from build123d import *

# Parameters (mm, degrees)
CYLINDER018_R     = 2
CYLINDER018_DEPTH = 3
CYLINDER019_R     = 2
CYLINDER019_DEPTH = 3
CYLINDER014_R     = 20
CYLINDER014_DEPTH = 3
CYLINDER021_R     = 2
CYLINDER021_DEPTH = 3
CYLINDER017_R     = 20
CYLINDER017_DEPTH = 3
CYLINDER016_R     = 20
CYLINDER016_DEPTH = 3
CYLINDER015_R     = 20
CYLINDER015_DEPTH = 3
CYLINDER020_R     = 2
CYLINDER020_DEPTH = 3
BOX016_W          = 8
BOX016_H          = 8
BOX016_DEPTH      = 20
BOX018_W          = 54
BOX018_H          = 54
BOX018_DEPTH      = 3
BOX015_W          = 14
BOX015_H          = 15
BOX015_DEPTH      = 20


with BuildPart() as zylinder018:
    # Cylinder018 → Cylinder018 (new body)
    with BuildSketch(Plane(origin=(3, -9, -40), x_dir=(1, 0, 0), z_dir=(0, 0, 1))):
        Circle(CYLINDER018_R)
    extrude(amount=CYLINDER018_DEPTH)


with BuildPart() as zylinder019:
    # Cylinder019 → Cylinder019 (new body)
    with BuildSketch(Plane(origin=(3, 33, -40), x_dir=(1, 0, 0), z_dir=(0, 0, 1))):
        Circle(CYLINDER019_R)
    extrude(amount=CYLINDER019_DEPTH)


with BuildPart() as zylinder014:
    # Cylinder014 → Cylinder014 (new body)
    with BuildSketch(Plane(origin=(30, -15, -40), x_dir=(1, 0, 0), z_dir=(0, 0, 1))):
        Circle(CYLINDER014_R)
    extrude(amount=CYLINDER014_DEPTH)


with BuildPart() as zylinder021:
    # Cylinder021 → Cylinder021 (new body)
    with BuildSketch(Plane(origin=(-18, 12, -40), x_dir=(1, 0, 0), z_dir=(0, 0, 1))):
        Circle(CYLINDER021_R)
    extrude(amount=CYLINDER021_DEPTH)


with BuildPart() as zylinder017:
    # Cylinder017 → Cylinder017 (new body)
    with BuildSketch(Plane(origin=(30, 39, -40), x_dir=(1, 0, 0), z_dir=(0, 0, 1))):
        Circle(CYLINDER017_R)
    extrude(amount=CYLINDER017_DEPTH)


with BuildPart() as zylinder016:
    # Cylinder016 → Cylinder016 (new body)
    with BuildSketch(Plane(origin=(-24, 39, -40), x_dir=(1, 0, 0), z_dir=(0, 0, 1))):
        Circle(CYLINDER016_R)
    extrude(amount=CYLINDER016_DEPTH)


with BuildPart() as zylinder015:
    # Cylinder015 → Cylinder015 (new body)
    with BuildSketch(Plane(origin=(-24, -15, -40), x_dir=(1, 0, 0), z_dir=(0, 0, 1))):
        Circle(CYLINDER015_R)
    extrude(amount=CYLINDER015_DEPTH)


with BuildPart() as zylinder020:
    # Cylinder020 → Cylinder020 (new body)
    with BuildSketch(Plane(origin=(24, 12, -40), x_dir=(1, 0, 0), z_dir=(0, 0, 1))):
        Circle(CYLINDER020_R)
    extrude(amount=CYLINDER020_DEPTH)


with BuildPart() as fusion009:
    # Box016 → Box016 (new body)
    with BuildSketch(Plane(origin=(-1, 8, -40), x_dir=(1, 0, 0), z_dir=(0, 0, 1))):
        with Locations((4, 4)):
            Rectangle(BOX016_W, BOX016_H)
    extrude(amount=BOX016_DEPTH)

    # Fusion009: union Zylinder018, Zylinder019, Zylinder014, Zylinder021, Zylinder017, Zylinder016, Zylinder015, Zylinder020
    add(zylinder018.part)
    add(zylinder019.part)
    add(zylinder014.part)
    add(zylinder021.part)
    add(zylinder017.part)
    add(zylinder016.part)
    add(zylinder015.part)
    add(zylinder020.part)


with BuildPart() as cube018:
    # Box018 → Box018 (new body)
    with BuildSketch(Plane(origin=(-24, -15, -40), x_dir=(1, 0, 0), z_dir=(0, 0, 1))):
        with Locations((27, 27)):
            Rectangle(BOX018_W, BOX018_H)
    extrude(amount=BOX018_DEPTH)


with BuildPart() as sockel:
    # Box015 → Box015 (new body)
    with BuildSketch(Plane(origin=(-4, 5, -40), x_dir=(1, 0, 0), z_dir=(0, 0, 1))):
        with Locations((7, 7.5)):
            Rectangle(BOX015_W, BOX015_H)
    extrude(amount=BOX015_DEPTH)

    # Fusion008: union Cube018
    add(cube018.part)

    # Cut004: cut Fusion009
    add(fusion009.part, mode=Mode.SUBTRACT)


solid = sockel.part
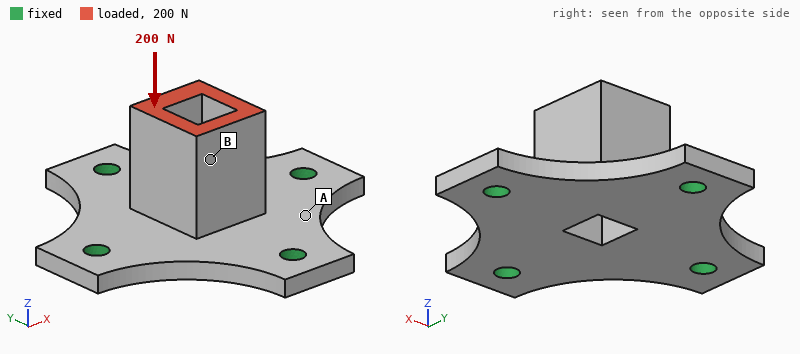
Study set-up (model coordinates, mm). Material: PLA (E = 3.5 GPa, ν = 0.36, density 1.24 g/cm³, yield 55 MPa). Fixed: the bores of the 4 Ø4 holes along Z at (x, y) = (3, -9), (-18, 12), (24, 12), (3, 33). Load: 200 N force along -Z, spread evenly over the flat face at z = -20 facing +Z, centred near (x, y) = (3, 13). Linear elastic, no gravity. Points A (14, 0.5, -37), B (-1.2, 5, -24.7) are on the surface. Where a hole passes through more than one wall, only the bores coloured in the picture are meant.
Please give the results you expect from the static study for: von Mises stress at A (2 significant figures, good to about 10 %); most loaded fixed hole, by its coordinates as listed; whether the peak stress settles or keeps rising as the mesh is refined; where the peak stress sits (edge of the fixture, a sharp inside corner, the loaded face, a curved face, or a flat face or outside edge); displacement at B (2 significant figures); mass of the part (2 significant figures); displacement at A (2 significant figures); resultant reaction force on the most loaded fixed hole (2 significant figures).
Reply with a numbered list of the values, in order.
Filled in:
1. 4.7 MPa
2. (3, 33)
3. keeps rising
4. edge of the fixture
5. 0.10 mm
6. 8.8 g
7. 0.046 mm
8. 59 N
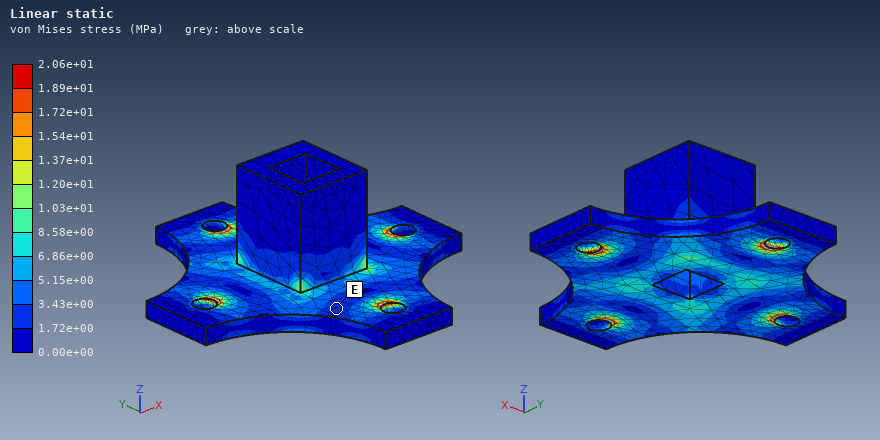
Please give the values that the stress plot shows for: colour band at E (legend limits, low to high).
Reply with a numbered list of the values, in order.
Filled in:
1. 1.72e+00 to 3.43e+00 MPa
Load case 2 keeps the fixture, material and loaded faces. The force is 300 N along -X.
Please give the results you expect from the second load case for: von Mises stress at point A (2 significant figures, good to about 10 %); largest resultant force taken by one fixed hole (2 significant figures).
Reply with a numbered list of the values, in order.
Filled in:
1. 13 MPa
2. 200 N
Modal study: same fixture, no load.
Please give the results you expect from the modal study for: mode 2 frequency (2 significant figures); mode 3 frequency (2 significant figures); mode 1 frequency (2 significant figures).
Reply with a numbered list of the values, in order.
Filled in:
1. 3200 Hz
2. 3300 Hz
3. 3200 Hz
